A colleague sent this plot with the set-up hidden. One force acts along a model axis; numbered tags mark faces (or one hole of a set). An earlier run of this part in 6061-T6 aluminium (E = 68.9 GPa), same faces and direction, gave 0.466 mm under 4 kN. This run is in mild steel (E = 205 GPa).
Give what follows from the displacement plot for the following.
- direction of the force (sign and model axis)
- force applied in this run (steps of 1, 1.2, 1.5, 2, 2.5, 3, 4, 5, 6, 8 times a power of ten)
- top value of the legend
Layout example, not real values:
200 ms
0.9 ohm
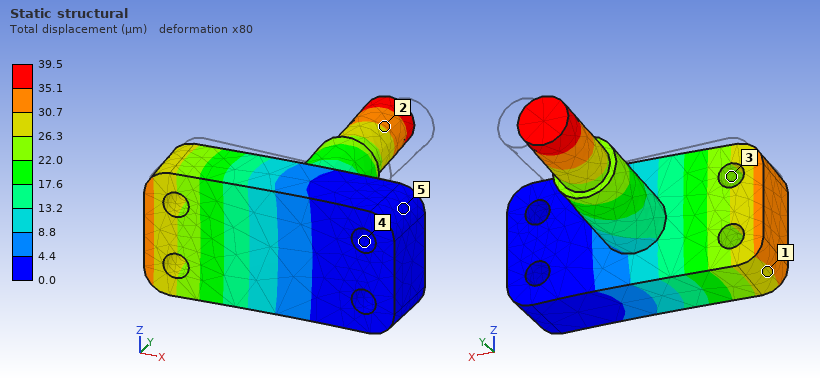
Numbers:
-Y
1 kN
39.5 µm
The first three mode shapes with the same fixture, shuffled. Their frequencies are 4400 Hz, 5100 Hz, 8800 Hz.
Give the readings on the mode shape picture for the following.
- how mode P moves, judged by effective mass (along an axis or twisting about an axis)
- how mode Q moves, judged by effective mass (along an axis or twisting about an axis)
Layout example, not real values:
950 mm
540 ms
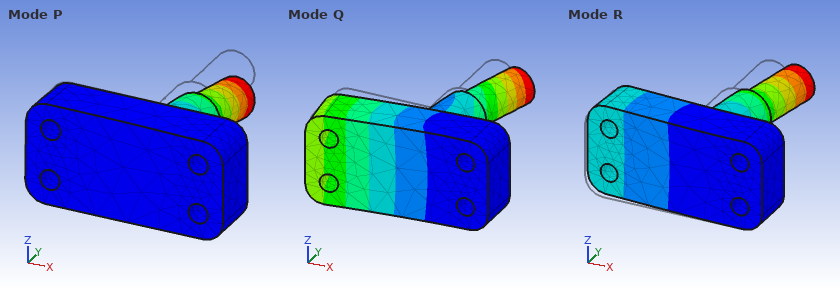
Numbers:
along Z
along Y
